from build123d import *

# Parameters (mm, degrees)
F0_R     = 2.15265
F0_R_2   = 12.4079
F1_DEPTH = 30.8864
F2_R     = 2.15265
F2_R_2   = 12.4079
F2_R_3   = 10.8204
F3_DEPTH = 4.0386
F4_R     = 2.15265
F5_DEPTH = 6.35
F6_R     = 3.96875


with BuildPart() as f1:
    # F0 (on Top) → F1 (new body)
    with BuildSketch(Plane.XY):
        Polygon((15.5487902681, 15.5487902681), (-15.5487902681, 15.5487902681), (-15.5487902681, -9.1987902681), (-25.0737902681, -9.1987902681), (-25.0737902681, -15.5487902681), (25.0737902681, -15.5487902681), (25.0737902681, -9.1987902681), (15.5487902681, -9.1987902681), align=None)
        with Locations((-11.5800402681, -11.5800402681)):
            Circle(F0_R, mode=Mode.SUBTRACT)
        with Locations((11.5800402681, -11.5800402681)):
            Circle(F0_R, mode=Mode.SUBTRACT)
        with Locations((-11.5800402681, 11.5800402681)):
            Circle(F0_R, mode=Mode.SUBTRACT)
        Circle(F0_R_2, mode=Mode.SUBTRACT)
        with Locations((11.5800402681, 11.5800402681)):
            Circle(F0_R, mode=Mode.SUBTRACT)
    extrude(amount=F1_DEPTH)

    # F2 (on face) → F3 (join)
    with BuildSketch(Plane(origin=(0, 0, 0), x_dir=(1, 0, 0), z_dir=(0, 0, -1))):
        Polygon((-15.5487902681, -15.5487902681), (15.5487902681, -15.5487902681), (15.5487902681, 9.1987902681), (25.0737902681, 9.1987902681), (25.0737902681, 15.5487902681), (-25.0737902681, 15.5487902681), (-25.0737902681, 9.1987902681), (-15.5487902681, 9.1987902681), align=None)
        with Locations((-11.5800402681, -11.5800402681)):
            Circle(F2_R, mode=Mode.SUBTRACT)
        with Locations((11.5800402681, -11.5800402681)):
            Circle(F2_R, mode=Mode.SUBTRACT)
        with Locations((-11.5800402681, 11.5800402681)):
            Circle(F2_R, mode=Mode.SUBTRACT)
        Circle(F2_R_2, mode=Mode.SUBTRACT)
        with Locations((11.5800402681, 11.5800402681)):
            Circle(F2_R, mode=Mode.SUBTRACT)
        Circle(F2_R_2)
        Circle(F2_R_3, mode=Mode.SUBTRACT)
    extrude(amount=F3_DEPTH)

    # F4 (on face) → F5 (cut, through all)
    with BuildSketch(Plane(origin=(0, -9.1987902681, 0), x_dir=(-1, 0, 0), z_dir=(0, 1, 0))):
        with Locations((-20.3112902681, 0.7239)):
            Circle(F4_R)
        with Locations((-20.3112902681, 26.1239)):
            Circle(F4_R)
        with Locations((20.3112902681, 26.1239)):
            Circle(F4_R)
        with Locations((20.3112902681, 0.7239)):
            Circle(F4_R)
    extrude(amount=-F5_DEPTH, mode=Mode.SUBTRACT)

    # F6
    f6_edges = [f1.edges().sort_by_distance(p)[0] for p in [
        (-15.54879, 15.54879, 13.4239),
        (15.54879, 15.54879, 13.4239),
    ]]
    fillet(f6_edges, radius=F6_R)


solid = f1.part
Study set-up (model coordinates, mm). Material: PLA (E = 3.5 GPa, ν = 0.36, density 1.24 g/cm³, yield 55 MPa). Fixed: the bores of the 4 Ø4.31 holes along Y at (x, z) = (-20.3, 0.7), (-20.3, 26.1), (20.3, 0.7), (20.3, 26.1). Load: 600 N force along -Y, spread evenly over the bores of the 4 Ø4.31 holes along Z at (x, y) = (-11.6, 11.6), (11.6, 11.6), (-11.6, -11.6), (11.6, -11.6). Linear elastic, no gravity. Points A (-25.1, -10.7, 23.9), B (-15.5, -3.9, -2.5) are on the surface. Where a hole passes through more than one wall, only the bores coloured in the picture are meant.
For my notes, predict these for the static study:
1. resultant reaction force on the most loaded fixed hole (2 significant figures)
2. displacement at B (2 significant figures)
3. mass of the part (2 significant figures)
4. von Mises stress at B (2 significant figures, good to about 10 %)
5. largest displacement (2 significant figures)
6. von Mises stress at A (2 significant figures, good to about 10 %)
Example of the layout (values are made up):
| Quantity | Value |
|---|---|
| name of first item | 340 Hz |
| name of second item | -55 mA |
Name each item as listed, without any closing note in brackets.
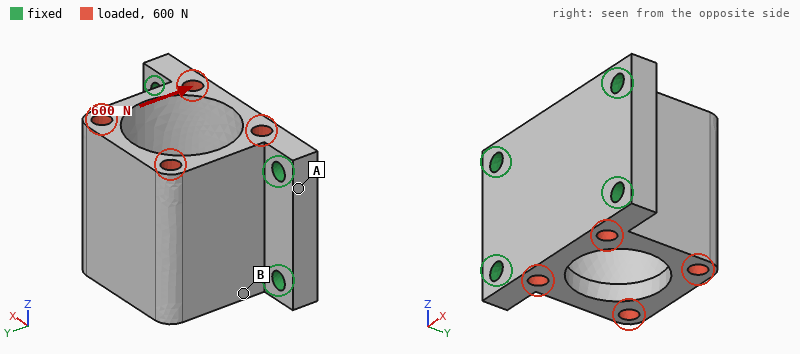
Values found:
| Quantity | Value |
|---|---|
| resultant reaction force on the most loaded fixed hole | 150 N |
| displacement at B | 23 µm |
| mass of the part | 23 g |
| von Mises stress at B | 4.0 MPa |
| largest displacement | 40 µm |
| von Mises stress at A | 1.5 MPa |
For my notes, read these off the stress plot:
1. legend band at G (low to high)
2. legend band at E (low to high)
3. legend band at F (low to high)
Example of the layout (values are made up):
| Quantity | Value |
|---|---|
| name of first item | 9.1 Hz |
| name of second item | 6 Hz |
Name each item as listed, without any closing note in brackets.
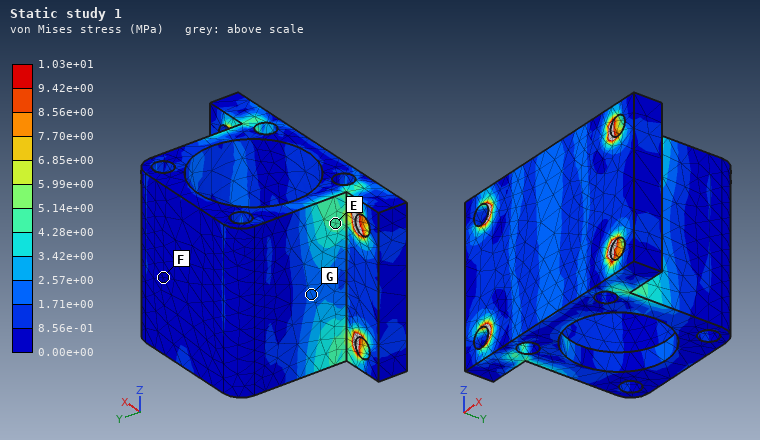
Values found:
| Quantity | Value |
|---|---|
| legend band at G | 1.71e+00 to 2.57e+00 MPa |
| legend band at E | 4.28e+00 to 5.14e+00 MPa |
| legend band at F | 0.00e+00 to 8.56e-01 MPa |
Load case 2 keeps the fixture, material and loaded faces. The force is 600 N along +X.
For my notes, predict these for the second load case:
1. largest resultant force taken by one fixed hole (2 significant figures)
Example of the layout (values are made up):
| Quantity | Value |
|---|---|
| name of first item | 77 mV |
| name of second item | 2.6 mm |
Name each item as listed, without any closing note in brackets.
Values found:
| Quantity | Value |
|---|---|
| largest resultant force taken by one fixed hole | 200 N |
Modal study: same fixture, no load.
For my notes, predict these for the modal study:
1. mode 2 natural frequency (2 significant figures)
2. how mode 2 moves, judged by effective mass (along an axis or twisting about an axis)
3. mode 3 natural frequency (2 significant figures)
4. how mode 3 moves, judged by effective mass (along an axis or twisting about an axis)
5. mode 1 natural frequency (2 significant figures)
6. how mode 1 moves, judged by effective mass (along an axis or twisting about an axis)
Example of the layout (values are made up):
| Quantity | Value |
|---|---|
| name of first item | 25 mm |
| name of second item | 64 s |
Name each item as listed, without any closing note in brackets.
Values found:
| Quantity | Value |
|---|---|
| mode 2 natural frequency | 3500 Hz |
| how mode 2 moves, judged by effective mass | along Z |
| mode 3 natural frequency | 4400 Hz |
| how mode 3 moves, judged by effective mass | twisting about Y |
| mode 1 natural frequency | 2400 Hz |
| how mode 1 moves, judged by effective mass | along X |
